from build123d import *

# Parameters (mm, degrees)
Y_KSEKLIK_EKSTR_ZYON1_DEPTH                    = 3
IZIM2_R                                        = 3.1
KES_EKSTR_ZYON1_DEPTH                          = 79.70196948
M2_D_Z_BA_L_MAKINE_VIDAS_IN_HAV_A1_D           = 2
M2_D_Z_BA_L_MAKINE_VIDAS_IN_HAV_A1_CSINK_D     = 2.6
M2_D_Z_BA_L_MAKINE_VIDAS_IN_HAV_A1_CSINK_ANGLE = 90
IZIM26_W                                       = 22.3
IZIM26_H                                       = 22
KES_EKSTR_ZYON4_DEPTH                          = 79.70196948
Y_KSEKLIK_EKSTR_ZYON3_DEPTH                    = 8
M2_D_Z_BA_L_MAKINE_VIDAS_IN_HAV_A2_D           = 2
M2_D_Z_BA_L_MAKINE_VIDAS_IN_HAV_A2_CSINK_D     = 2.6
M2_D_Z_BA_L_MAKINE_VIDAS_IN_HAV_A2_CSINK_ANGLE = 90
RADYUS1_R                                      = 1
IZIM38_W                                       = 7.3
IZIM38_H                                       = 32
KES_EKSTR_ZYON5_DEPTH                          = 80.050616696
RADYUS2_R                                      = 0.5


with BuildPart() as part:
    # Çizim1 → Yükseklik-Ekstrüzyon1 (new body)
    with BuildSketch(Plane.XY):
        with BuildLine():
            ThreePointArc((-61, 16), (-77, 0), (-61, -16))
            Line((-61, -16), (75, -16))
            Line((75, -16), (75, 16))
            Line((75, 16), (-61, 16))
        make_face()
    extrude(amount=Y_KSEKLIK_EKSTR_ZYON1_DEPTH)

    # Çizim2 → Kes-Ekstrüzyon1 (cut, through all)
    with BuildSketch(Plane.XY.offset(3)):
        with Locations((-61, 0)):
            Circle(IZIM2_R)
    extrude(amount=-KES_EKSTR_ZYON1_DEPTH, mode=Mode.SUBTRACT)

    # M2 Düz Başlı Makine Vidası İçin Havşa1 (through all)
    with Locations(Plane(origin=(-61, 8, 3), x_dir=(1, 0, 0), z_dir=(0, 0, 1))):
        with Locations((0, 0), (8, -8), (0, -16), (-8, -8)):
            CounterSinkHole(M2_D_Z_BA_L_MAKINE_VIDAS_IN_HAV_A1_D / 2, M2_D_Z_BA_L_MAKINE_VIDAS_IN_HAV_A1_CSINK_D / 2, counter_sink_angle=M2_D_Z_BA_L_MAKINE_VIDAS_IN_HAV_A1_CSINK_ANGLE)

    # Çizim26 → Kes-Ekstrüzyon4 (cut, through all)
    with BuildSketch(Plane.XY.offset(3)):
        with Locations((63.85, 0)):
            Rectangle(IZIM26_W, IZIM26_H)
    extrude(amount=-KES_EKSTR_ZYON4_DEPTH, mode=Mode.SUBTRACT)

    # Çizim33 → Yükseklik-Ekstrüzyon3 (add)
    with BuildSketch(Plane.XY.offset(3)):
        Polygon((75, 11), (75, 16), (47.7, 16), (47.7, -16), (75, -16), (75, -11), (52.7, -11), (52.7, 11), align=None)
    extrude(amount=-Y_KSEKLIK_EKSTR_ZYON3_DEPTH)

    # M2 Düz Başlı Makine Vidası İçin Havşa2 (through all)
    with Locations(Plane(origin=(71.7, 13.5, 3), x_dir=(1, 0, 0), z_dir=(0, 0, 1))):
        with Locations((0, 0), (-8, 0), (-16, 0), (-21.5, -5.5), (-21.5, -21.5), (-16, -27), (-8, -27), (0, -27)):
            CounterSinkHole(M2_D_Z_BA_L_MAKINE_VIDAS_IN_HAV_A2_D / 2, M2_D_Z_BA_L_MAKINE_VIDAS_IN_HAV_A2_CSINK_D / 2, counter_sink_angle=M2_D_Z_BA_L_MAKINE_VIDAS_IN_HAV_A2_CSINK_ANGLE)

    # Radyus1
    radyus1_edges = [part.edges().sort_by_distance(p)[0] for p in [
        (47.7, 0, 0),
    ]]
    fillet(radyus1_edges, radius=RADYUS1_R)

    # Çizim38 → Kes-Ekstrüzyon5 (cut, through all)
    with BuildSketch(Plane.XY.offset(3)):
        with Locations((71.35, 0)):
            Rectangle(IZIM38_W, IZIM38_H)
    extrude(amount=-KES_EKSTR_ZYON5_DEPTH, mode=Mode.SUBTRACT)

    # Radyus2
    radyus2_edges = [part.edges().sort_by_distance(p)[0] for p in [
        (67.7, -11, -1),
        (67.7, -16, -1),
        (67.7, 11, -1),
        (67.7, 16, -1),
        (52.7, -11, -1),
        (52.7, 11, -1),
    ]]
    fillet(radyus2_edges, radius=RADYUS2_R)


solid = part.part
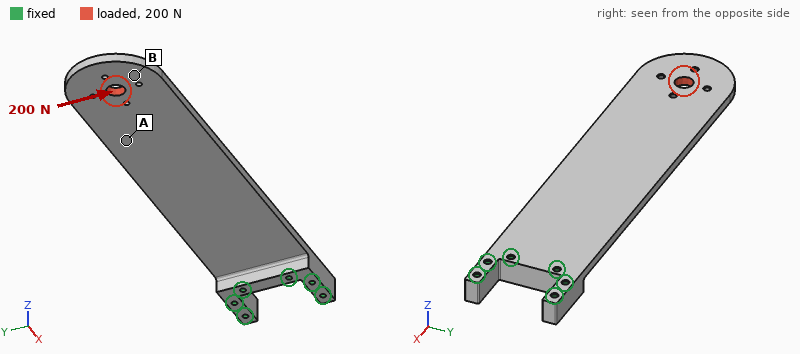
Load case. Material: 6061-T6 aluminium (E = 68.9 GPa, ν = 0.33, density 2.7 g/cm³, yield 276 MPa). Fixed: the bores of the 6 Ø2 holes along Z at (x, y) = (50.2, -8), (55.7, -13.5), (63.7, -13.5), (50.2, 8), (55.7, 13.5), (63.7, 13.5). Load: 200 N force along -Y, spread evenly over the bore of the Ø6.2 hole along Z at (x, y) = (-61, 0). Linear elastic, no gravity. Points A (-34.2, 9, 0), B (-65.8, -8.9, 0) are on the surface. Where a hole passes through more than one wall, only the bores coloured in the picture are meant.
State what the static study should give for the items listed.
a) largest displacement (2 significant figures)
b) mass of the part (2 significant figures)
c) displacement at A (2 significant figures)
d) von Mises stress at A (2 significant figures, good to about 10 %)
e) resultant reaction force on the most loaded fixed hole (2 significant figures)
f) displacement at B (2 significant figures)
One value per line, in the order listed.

0.22 mm
37 g
0.12 mm
6.9 MPa
540 N
0.19 mm
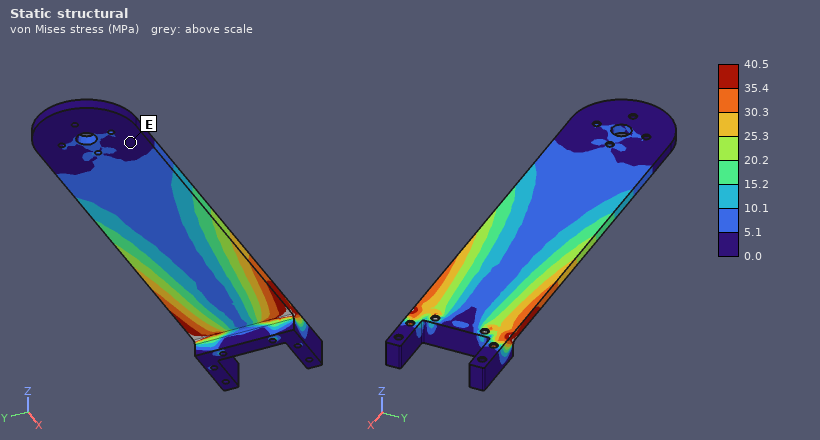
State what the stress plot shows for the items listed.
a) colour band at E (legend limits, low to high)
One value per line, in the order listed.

0.0 to 5.1 MPa
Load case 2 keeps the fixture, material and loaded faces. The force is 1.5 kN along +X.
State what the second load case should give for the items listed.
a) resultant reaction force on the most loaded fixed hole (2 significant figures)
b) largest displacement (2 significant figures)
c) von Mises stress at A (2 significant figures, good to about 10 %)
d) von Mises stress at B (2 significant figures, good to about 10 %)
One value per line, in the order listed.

540 N
47 µm
16 MPa
9.6 MPa
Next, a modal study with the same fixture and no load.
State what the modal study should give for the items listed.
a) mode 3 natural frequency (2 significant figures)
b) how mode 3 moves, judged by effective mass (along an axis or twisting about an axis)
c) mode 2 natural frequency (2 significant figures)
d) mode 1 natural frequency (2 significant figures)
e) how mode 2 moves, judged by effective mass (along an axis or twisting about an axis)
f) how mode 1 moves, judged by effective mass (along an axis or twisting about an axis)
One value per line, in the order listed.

1300 Hz
twisting about X
1000 Hz
170 Hz
along Z
along Z
